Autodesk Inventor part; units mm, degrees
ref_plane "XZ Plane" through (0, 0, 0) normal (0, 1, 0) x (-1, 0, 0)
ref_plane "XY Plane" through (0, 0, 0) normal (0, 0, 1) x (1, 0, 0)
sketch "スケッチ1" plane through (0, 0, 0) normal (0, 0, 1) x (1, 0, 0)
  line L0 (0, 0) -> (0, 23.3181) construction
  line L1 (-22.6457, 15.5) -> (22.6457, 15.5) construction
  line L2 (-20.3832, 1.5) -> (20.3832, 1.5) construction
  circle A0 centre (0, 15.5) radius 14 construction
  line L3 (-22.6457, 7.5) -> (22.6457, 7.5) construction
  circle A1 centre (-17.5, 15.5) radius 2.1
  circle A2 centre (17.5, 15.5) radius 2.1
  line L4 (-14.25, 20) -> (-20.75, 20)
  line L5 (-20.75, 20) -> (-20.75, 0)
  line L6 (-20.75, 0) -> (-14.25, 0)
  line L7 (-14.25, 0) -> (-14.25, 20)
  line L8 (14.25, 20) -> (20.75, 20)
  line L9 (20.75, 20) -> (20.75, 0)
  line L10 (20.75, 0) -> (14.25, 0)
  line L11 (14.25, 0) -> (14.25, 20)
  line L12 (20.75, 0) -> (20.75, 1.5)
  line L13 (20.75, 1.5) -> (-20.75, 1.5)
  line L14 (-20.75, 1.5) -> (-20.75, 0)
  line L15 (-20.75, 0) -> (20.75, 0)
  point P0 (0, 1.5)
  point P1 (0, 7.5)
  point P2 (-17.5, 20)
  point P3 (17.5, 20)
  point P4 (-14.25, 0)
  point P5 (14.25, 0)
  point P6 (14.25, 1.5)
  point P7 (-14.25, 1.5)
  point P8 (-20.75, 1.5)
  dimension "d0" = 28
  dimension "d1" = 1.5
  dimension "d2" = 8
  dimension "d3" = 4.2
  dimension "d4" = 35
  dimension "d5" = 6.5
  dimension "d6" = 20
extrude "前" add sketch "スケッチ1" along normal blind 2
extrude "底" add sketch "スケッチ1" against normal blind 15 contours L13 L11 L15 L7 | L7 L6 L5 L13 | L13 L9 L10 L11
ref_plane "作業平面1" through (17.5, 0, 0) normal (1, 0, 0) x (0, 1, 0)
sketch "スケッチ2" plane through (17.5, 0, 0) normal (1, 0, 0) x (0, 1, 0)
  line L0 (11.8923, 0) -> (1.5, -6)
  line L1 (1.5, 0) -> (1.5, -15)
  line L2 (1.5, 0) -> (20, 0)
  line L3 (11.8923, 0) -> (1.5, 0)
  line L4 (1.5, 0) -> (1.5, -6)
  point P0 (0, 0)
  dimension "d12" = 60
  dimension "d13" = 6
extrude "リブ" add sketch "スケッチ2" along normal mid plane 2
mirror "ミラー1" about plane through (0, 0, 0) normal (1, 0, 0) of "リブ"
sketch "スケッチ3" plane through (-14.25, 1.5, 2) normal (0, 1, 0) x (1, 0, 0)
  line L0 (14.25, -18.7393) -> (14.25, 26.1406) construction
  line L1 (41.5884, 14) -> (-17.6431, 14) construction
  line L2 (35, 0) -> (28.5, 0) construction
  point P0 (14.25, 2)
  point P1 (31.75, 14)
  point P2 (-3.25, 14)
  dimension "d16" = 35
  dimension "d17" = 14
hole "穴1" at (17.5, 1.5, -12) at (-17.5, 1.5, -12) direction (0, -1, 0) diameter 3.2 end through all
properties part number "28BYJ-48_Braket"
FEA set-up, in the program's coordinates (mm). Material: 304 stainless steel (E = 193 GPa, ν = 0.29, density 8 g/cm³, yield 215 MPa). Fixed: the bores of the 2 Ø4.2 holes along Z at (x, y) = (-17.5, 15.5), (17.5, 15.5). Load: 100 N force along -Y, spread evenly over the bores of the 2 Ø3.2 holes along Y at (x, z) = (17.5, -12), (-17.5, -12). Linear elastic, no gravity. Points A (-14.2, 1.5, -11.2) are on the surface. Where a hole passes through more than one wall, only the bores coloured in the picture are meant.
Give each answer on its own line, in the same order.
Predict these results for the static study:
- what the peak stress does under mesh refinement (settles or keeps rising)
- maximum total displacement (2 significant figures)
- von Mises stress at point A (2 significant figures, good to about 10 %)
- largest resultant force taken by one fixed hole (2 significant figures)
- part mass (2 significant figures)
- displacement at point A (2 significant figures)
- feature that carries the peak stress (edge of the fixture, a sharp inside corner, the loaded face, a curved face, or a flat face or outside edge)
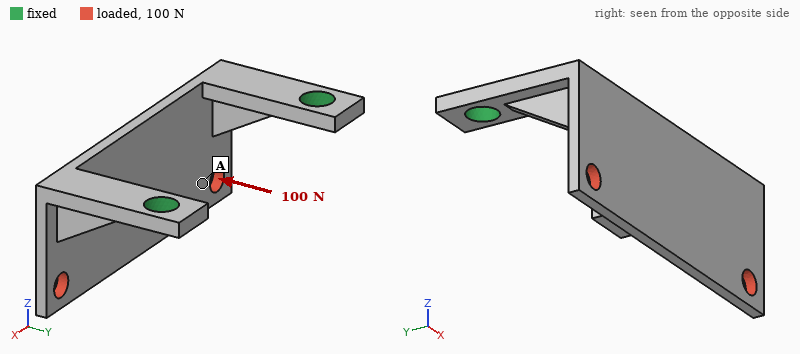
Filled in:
keeps rising
93 µm
28 MPa
50 N
13 g
67 µm
edge of the fixture
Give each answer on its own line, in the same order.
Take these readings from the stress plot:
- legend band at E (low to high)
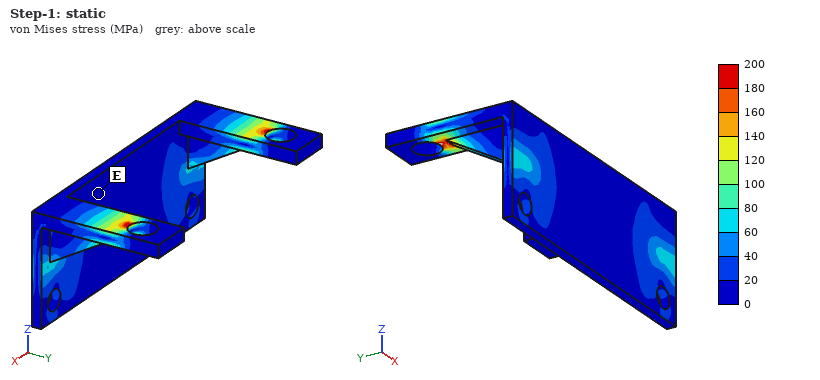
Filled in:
0 to 20 MPa
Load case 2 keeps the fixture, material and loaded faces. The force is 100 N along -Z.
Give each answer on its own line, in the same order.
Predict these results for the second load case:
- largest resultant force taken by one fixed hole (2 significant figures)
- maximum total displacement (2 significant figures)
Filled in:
50 N
59 µm
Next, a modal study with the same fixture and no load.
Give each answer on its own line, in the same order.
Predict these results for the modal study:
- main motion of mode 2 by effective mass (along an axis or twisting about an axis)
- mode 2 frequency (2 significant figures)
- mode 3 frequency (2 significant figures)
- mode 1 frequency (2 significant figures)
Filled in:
along X
3800 Hz
5400 Hz
2200 Hz
